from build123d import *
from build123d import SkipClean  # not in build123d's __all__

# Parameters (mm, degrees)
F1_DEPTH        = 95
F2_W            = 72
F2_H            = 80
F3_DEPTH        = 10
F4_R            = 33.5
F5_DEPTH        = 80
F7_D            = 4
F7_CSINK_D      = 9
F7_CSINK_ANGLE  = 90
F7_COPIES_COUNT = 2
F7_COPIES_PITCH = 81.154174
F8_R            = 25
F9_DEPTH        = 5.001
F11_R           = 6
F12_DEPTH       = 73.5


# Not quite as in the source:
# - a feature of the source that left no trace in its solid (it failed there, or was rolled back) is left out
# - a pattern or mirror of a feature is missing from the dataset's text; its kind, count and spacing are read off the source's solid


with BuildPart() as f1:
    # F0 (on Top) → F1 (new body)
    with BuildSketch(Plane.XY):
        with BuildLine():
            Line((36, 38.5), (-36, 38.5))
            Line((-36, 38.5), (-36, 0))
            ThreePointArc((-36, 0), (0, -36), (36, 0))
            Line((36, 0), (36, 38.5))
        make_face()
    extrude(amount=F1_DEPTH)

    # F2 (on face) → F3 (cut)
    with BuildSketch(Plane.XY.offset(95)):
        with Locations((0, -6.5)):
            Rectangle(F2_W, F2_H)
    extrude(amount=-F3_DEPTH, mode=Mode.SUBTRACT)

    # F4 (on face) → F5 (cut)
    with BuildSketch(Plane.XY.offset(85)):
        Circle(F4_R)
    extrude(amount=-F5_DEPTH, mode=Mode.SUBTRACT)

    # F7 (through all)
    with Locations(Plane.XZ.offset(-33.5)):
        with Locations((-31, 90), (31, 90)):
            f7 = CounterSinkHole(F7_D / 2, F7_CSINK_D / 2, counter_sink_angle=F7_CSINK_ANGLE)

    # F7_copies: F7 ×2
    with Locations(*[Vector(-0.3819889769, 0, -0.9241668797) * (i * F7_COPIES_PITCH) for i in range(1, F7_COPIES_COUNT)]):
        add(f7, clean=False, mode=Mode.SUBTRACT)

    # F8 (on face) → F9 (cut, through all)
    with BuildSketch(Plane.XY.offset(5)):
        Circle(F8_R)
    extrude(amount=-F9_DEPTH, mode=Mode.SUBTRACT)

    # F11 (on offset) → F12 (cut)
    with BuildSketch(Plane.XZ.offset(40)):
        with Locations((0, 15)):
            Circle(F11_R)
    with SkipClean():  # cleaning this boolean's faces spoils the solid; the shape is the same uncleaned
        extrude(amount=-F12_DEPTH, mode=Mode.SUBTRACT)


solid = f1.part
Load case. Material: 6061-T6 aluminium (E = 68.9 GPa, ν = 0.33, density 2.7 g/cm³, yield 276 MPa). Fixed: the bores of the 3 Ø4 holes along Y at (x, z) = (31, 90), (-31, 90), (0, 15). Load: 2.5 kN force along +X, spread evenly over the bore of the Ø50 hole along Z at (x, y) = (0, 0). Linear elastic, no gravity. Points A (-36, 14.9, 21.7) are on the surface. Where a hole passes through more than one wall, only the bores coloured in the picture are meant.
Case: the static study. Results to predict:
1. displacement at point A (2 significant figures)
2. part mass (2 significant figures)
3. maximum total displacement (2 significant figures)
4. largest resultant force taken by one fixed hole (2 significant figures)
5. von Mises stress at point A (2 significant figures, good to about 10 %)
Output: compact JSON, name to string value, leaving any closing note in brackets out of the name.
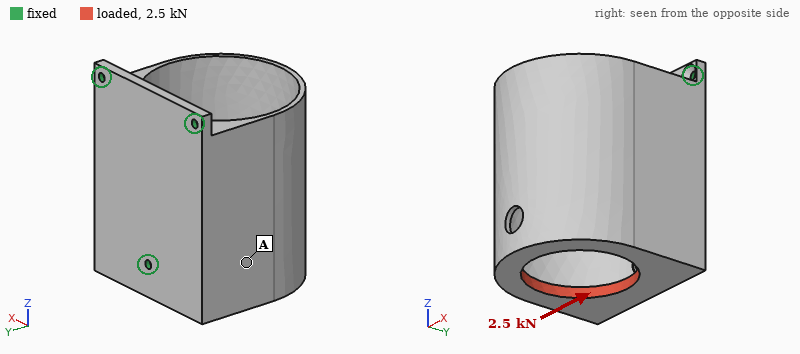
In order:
{"displacement at point A": "0.11 mm", "part mass": "320 g", "maximum total displacement": "0.39 mm", "largest resultant force taken by one fixed hole": "2.2 kN", "von Mises stress at point A": "12 MPa"}
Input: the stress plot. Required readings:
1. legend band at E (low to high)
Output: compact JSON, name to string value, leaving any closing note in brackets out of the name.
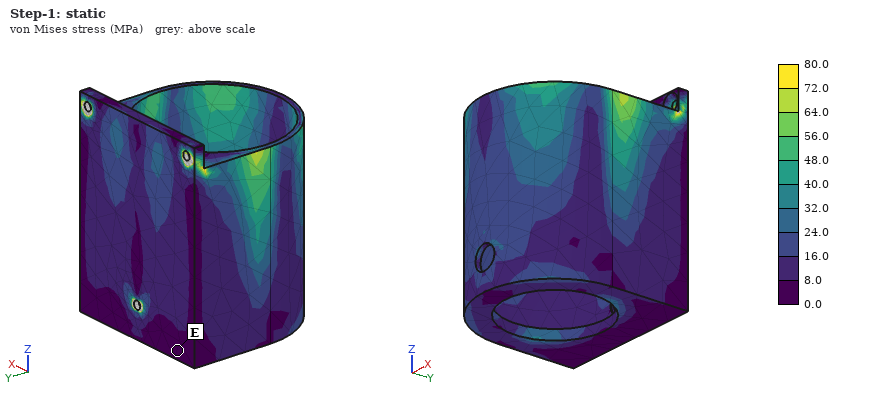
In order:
{"legend band at E": "0.0 to 8.0 MPa"}
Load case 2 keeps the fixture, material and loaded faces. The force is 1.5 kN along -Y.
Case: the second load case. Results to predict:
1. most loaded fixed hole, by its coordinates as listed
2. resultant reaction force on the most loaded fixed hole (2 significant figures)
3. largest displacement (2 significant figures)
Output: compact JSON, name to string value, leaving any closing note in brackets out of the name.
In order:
{"most loaded fixed hole, by its coordinates as listed": "(0, 15)", "resultant reaction force on the most loaded fixed hole": "1.7 kN", "largest displacement": "74 µm"}
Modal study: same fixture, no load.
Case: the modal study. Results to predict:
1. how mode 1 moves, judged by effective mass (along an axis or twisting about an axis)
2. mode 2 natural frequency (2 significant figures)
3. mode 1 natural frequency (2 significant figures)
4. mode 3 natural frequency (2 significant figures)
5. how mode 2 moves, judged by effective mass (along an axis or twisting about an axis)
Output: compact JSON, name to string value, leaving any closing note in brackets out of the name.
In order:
{"how mode 1 moves, judged by effective mass": "along X", "mode 2 natural frequency": "2200 Hz", "mode 1 natural frequency": "1100 Hz", "mode 3 natural frequency": "2800 Hz", "how mode 2 moves, judged by effective mass": "along Y"}
